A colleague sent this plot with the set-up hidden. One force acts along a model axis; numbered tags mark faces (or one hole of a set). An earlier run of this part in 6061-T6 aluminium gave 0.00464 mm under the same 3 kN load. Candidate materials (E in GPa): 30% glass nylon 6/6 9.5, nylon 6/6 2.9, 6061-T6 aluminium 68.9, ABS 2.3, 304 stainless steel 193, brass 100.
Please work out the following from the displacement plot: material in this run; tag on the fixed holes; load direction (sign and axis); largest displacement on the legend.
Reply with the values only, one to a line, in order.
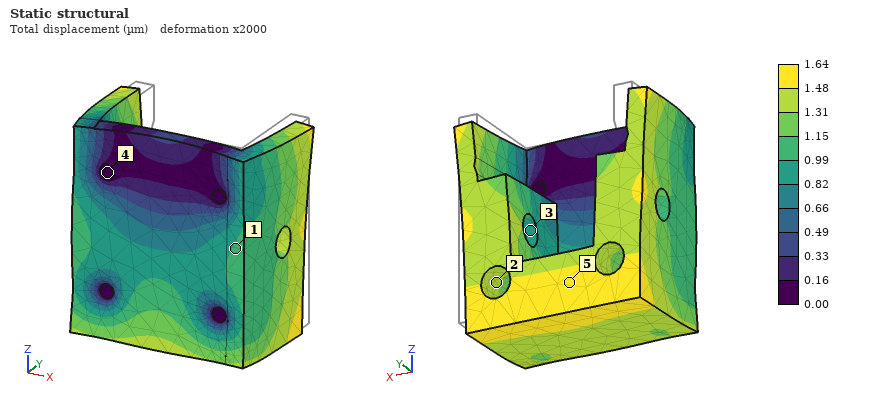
304 stainless steel
4
-Y
1.64 µm
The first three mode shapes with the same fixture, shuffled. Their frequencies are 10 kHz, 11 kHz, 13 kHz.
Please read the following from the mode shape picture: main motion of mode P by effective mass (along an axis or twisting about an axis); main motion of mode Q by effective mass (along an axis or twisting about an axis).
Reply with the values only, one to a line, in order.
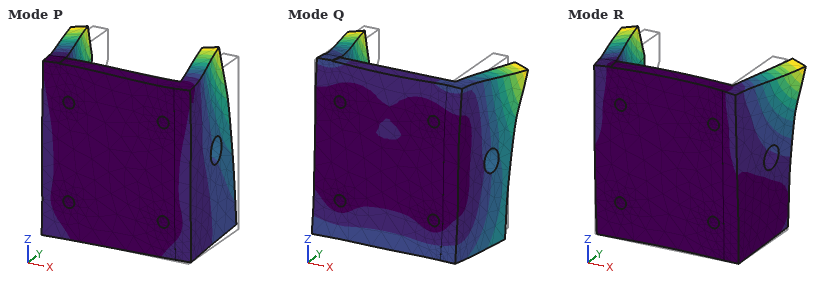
along X
along Z
